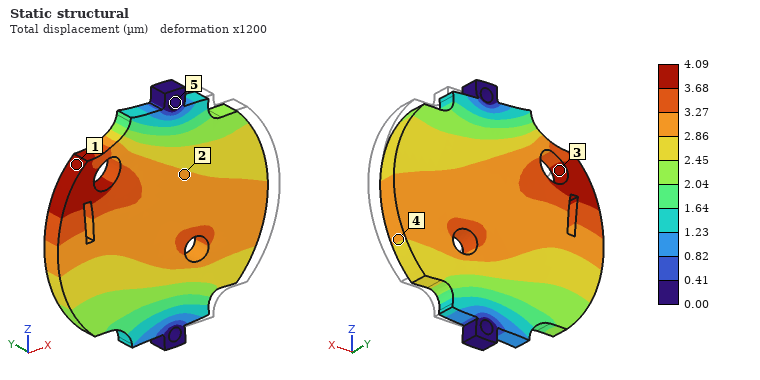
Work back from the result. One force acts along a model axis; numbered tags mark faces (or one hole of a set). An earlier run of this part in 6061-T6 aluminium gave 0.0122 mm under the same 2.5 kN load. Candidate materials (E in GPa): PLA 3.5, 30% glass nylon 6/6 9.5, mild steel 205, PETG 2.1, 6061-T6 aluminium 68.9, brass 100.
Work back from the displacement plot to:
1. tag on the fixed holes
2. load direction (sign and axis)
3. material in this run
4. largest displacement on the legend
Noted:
5
-X
mild steel
4.09 µm
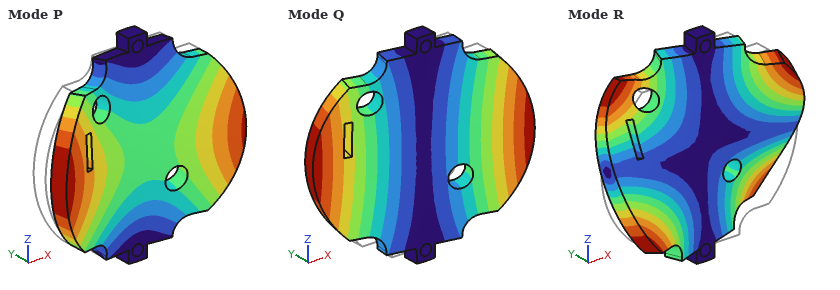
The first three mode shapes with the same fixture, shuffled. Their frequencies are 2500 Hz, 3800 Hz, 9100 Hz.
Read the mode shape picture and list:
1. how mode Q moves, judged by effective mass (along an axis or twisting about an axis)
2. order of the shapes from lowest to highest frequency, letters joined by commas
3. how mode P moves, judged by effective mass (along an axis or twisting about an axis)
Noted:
twisting about Z
Q, P, R
along Y
